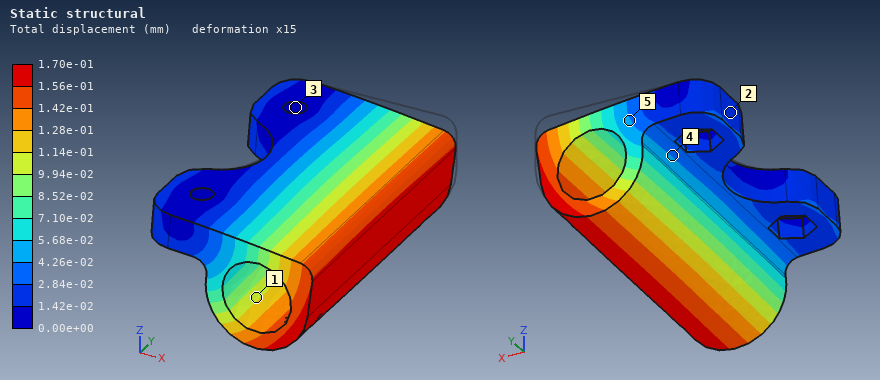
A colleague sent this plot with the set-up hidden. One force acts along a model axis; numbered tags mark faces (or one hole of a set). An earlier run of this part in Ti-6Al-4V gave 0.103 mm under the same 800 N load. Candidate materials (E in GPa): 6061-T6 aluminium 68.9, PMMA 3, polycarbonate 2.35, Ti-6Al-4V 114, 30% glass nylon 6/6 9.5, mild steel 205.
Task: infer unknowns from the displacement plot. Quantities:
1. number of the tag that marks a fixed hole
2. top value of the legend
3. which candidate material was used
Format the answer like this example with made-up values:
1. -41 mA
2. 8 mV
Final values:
1. 3
2. 1.70e-01 mm
3. 6061-T6 aluminium
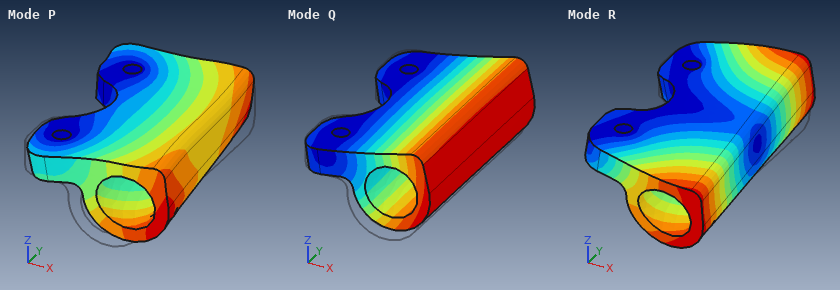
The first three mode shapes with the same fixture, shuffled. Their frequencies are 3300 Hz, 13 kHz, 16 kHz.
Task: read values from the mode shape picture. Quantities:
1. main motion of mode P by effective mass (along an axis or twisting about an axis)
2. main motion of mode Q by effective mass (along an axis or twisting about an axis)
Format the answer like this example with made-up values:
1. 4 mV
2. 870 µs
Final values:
1. along Y
2. along Z
